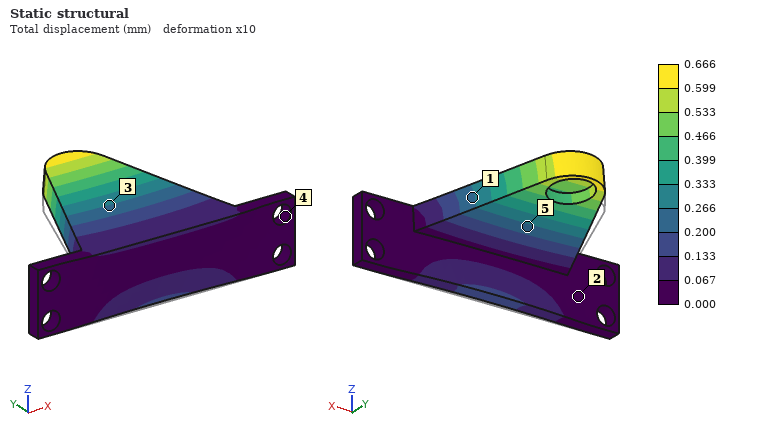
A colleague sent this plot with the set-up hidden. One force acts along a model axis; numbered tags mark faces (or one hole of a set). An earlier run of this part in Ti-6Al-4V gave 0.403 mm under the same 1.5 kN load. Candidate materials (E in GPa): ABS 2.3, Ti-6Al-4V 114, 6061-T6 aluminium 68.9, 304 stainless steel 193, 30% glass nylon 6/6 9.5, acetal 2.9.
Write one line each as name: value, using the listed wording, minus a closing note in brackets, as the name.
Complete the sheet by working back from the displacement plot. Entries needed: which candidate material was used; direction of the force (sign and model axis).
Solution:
which candidate material was used: 6061-T6 aluminium
direction of the force: +Z
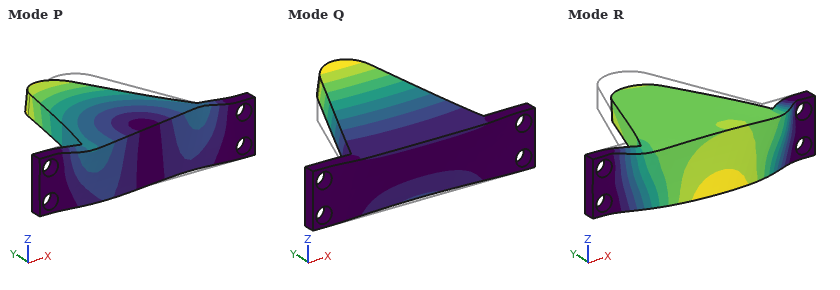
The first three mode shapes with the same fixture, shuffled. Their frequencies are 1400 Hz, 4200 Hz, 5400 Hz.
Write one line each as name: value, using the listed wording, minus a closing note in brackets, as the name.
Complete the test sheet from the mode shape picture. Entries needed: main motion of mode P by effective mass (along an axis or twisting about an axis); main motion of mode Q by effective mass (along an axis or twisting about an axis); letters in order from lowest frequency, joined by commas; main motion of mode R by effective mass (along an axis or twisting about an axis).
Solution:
main motion of mode P by effective mass: along X
main motion of mode Q by effective mass: along Z
letters in order from lowest frequency, joined by commas: Q, R, P
main motion of mode R by effective mass: along Y
